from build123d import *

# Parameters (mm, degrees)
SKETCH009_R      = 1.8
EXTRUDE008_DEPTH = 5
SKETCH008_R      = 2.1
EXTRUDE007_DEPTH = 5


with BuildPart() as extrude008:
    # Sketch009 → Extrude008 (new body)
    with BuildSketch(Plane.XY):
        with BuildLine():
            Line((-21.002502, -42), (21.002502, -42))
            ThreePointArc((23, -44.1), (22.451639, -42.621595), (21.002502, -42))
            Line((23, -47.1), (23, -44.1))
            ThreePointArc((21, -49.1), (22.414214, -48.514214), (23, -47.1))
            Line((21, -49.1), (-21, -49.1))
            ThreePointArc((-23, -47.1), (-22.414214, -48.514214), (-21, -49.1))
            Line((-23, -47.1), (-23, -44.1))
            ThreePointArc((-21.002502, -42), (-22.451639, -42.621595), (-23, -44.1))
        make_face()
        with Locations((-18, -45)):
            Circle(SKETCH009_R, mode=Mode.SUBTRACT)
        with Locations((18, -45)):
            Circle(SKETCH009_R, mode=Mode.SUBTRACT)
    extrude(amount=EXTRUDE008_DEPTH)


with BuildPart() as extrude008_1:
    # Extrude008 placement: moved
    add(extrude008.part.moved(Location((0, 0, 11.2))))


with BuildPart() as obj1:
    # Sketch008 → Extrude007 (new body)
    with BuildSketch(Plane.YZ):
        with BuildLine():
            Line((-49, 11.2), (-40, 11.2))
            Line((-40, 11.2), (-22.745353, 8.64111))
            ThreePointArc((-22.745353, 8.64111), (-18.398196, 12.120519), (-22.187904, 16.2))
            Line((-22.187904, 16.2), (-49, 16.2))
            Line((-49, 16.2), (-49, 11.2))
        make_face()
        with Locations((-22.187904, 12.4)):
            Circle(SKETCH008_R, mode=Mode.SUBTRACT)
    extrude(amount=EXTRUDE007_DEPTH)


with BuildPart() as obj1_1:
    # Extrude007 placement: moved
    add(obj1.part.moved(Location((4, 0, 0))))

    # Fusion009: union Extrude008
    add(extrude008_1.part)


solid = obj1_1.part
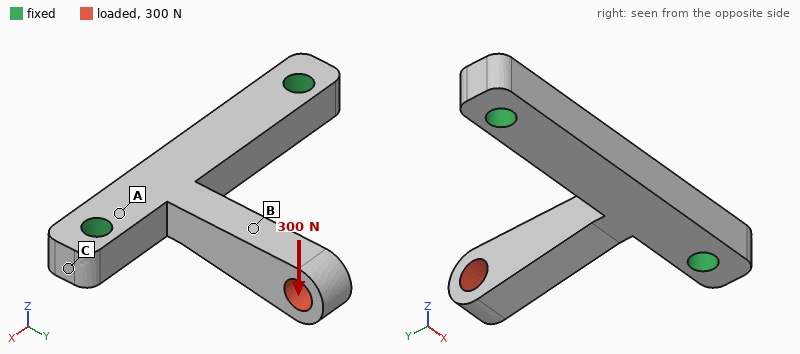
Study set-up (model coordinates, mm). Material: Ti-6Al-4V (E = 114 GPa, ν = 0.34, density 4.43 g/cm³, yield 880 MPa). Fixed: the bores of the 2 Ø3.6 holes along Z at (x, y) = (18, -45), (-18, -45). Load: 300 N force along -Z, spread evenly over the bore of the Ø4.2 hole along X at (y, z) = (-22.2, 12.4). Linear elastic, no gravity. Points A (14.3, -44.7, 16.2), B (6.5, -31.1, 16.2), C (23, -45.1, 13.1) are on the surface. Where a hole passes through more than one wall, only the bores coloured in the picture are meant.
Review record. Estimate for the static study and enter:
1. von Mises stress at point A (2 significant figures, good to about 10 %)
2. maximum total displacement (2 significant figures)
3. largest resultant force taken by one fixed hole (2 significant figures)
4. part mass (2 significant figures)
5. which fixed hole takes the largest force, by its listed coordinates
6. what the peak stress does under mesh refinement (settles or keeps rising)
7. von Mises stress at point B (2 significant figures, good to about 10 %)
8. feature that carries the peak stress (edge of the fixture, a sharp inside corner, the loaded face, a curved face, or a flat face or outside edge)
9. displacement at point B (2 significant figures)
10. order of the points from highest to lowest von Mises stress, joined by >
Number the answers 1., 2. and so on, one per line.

1. 190 MPa
2. 0.37 mm
3. 250 N
4. 9.6 g
5. (18, -45)
6. keeps rising
7. 82 MPa
8. a sharp inside corner
9. 0.17 mm
10. A > B > C
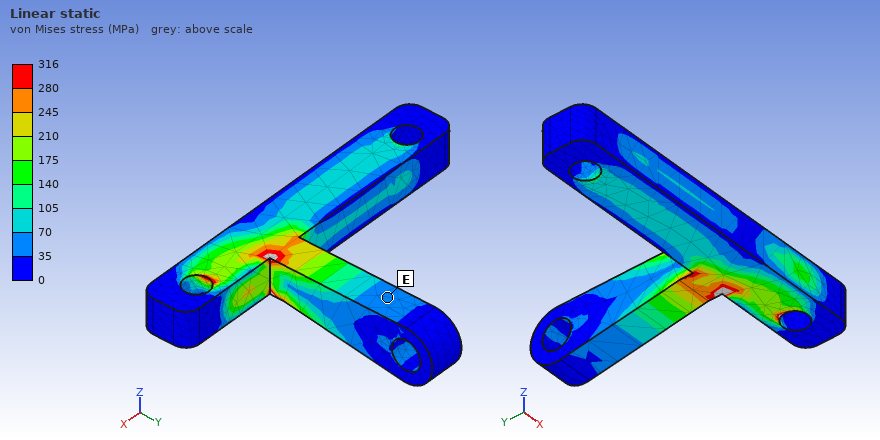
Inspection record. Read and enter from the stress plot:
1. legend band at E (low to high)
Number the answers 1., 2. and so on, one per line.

1. 35 to 70 MPa
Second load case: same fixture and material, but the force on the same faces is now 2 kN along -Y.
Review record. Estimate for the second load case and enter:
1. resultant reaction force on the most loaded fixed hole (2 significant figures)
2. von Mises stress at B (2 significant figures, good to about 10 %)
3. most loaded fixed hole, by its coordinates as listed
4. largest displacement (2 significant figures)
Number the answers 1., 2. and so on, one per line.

1. 1.5 kN
2. 24 MPa
3. (18, -45)
4. 0.16 mm
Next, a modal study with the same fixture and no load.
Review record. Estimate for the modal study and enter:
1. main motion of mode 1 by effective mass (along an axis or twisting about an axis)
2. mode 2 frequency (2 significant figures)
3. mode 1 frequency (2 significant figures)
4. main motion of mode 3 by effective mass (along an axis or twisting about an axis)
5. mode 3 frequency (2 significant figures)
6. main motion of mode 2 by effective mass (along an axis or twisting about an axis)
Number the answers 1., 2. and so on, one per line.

1. along Z
2. 5900 Hz
3. 4300 Hz
4. along Y
5. 18 kHz
6. along X
